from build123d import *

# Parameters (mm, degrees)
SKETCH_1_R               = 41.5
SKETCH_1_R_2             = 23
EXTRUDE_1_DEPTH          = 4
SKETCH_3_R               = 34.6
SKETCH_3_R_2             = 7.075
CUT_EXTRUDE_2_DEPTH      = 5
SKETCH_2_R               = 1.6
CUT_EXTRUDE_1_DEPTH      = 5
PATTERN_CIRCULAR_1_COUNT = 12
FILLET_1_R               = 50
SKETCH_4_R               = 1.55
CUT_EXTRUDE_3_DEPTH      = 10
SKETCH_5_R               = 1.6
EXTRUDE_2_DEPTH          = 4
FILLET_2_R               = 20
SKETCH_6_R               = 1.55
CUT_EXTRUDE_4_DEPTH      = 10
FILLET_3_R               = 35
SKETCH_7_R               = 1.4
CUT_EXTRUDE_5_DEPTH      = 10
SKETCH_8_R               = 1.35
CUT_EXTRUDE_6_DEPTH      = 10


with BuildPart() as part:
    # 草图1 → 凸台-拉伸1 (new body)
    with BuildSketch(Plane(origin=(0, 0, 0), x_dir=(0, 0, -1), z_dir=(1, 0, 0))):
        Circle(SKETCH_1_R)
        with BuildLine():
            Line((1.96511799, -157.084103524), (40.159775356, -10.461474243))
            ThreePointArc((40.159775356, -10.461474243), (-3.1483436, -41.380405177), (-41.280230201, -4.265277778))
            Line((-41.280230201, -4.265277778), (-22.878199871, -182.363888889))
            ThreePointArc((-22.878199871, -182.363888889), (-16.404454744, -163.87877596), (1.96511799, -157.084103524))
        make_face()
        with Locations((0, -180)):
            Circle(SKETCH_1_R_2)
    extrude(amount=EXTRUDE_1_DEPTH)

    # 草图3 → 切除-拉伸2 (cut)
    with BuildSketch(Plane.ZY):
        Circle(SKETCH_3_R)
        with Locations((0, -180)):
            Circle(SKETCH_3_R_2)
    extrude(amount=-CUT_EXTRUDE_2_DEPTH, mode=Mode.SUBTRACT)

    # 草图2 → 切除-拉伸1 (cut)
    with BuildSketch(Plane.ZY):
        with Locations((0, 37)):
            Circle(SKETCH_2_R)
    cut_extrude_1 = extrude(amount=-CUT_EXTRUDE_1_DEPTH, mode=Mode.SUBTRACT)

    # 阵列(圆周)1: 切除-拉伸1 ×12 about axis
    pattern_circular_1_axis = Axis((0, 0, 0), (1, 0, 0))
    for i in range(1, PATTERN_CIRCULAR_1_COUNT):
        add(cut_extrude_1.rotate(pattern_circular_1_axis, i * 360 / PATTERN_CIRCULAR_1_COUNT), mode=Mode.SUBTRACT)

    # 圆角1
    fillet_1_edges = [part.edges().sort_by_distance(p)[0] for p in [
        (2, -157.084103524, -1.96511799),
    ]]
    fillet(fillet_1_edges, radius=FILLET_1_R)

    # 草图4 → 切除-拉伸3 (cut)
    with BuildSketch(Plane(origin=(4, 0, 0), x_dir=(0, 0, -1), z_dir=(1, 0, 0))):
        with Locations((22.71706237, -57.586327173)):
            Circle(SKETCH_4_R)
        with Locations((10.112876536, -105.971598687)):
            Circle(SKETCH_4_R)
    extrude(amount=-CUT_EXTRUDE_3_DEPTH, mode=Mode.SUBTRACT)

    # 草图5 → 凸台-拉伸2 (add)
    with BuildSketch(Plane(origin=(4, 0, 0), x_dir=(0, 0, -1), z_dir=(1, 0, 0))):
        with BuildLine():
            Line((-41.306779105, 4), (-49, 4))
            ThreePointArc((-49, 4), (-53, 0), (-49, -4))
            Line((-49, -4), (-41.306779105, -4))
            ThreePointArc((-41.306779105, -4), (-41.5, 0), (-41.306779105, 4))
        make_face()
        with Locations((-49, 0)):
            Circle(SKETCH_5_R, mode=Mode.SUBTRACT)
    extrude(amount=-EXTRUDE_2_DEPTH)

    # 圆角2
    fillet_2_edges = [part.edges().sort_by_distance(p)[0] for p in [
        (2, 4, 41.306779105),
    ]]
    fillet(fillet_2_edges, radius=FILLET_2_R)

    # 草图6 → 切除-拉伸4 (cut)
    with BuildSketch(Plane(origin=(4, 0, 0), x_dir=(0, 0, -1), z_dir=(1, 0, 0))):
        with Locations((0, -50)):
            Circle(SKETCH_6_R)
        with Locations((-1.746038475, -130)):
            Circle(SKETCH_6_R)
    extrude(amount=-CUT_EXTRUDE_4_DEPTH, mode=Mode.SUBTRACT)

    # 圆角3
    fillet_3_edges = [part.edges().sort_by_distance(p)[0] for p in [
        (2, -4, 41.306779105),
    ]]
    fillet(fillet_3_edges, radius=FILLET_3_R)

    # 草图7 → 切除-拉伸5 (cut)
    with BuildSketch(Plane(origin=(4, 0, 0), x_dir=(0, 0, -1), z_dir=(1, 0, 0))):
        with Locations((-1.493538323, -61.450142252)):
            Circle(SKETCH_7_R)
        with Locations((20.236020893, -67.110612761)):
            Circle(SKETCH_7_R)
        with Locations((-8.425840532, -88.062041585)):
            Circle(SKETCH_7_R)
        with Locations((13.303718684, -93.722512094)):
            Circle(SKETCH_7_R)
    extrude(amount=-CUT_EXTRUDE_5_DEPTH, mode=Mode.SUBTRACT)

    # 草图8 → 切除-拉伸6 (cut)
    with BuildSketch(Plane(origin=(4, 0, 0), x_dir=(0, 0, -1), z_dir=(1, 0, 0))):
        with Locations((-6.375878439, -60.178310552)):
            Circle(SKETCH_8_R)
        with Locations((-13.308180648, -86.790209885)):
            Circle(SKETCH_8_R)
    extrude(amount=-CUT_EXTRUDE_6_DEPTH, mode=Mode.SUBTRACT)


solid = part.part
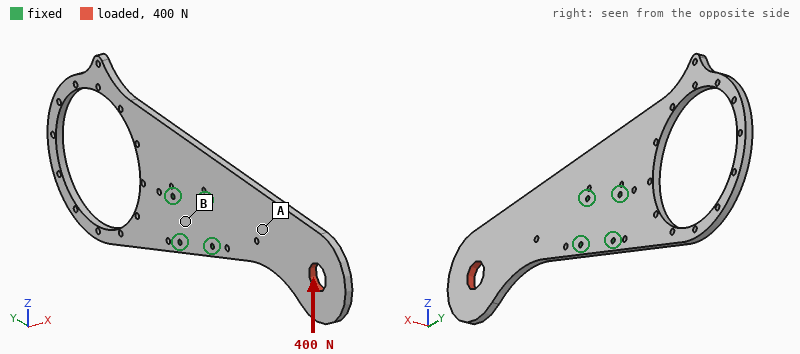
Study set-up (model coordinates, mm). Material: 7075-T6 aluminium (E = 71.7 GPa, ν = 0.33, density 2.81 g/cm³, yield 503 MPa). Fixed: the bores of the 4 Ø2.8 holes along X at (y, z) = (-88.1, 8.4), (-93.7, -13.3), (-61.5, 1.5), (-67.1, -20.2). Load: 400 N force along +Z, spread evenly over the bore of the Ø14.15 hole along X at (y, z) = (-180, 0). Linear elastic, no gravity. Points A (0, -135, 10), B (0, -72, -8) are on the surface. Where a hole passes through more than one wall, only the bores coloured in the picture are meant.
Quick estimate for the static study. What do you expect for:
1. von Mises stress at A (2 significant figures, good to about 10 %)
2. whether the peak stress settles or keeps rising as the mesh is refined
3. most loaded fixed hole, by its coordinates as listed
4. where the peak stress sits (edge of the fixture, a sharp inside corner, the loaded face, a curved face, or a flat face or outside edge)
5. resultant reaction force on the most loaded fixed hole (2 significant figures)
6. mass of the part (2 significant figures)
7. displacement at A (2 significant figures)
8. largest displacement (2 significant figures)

5.7 MPa
keeps rising
(-93.7, -13.3)
edge of the fixture
1.0 kN
110 g
0.024 mm
0.10 mm
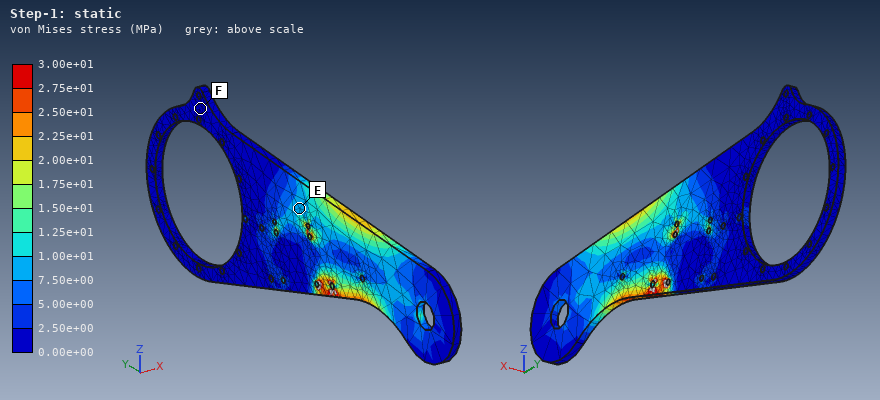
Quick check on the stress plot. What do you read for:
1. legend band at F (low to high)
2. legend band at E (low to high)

0.00e+00 to 2.50e+00 MPa
7.50e+00 to 1.00e+01 MPa
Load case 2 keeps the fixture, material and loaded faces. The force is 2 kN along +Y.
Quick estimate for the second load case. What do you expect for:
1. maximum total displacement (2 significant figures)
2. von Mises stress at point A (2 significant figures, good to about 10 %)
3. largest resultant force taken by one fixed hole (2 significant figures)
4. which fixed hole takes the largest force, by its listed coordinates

62 µm
12 MPa
940 N
(-88.1, 8.4)
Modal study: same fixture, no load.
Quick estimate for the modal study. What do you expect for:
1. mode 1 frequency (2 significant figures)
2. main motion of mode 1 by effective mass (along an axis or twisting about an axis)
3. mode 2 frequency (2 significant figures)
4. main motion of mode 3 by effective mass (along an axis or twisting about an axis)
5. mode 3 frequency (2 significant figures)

280 Hz
along X
360 Hz
twisting about Y
730 Hz
